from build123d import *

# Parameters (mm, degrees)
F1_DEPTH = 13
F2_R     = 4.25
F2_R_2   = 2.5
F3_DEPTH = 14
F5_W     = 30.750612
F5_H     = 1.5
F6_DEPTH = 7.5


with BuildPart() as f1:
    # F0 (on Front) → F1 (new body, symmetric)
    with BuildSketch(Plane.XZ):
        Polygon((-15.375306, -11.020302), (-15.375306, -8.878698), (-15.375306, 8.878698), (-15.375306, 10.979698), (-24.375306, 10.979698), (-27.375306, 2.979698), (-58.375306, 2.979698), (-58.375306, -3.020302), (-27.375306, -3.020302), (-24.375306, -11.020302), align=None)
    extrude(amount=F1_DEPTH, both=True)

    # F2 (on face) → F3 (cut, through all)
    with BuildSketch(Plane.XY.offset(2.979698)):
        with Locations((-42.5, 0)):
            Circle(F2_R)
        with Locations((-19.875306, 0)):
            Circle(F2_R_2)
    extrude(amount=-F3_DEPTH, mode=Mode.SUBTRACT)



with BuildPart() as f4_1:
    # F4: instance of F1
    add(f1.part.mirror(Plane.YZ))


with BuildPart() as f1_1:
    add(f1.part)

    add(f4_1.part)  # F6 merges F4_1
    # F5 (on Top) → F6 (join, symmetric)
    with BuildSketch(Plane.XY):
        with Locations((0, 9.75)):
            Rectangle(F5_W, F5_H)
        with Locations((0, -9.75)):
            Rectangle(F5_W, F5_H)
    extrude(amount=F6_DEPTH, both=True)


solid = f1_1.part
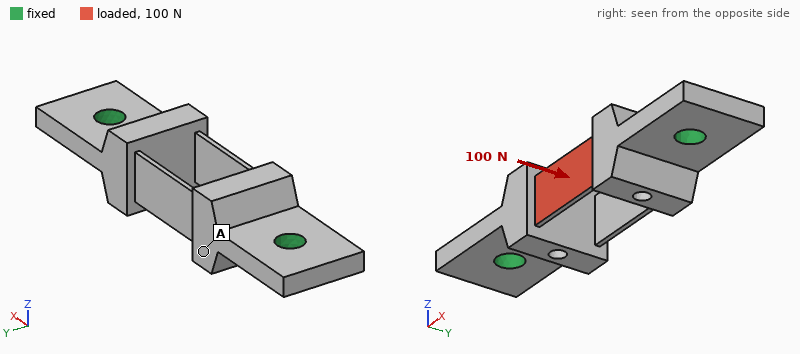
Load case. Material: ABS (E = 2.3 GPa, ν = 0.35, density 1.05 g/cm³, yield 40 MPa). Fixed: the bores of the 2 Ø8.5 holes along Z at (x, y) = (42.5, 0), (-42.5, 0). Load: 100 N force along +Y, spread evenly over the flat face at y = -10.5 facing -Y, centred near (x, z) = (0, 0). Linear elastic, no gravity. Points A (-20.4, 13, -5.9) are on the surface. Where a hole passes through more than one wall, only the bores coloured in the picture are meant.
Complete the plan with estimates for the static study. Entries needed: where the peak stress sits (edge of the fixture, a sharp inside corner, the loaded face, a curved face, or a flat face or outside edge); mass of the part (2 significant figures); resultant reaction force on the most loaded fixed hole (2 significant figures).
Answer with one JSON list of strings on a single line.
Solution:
["a flat face or outside edge", "23 g", "50 N"]
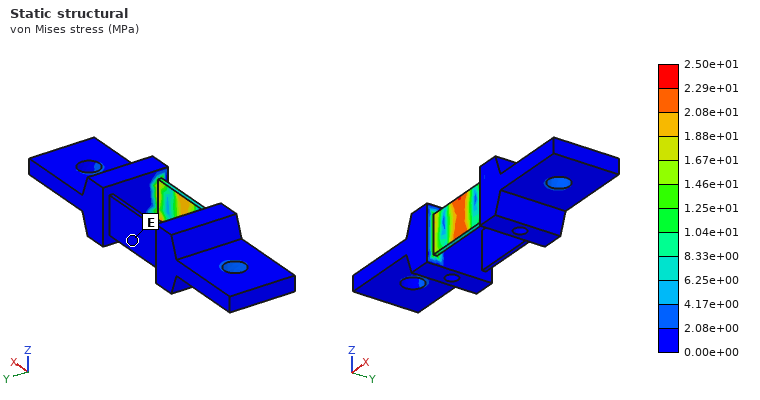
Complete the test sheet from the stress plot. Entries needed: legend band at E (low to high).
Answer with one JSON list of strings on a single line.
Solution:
["0.00e+00 to 2.08e+00 MPa"]
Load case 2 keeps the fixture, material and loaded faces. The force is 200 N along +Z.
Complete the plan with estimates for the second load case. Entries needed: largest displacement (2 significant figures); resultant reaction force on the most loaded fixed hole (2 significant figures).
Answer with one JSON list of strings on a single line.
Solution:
["0.57 mm", "100 N"]
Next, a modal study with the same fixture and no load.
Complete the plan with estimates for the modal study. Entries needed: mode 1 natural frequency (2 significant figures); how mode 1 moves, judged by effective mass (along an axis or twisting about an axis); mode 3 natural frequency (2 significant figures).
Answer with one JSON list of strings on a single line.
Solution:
["1500 Hz", "along Z", "2200 Hz"]
